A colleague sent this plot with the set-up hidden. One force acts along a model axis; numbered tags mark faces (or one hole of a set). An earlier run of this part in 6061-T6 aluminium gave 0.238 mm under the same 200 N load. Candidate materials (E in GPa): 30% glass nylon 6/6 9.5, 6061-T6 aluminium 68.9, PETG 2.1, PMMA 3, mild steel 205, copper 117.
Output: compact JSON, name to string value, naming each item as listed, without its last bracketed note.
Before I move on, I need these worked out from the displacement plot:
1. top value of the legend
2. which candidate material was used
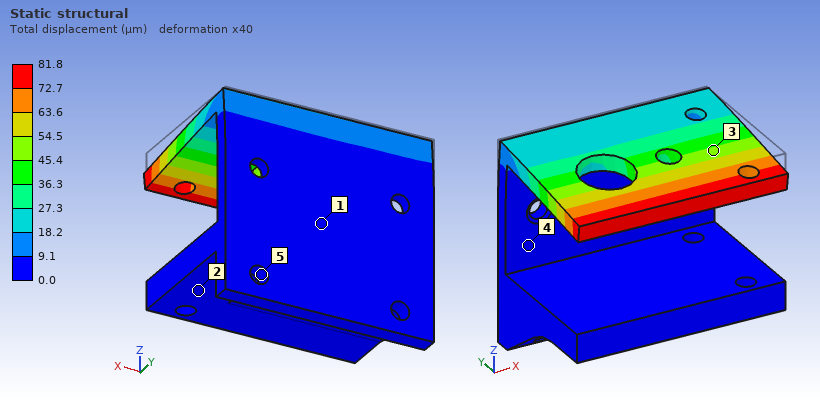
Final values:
{"top value of the legend": "81.8 µm", "which candidate material was used": "mild steel"}
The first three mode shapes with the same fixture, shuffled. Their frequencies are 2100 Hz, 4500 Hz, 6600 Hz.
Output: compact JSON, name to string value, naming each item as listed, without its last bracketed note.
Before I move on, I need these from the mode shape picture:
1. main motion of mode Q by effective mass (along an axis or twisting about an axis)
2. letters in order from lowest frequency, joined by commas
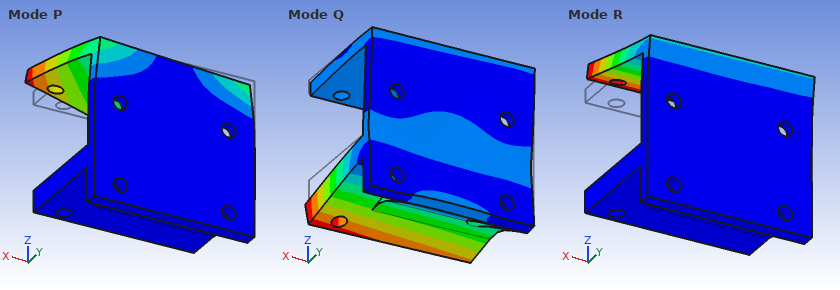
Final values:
{"main motion of mode Q by effective mass": "along Z", "letters in order from lowest frequency, joined by commas": "R, P, Q"}
